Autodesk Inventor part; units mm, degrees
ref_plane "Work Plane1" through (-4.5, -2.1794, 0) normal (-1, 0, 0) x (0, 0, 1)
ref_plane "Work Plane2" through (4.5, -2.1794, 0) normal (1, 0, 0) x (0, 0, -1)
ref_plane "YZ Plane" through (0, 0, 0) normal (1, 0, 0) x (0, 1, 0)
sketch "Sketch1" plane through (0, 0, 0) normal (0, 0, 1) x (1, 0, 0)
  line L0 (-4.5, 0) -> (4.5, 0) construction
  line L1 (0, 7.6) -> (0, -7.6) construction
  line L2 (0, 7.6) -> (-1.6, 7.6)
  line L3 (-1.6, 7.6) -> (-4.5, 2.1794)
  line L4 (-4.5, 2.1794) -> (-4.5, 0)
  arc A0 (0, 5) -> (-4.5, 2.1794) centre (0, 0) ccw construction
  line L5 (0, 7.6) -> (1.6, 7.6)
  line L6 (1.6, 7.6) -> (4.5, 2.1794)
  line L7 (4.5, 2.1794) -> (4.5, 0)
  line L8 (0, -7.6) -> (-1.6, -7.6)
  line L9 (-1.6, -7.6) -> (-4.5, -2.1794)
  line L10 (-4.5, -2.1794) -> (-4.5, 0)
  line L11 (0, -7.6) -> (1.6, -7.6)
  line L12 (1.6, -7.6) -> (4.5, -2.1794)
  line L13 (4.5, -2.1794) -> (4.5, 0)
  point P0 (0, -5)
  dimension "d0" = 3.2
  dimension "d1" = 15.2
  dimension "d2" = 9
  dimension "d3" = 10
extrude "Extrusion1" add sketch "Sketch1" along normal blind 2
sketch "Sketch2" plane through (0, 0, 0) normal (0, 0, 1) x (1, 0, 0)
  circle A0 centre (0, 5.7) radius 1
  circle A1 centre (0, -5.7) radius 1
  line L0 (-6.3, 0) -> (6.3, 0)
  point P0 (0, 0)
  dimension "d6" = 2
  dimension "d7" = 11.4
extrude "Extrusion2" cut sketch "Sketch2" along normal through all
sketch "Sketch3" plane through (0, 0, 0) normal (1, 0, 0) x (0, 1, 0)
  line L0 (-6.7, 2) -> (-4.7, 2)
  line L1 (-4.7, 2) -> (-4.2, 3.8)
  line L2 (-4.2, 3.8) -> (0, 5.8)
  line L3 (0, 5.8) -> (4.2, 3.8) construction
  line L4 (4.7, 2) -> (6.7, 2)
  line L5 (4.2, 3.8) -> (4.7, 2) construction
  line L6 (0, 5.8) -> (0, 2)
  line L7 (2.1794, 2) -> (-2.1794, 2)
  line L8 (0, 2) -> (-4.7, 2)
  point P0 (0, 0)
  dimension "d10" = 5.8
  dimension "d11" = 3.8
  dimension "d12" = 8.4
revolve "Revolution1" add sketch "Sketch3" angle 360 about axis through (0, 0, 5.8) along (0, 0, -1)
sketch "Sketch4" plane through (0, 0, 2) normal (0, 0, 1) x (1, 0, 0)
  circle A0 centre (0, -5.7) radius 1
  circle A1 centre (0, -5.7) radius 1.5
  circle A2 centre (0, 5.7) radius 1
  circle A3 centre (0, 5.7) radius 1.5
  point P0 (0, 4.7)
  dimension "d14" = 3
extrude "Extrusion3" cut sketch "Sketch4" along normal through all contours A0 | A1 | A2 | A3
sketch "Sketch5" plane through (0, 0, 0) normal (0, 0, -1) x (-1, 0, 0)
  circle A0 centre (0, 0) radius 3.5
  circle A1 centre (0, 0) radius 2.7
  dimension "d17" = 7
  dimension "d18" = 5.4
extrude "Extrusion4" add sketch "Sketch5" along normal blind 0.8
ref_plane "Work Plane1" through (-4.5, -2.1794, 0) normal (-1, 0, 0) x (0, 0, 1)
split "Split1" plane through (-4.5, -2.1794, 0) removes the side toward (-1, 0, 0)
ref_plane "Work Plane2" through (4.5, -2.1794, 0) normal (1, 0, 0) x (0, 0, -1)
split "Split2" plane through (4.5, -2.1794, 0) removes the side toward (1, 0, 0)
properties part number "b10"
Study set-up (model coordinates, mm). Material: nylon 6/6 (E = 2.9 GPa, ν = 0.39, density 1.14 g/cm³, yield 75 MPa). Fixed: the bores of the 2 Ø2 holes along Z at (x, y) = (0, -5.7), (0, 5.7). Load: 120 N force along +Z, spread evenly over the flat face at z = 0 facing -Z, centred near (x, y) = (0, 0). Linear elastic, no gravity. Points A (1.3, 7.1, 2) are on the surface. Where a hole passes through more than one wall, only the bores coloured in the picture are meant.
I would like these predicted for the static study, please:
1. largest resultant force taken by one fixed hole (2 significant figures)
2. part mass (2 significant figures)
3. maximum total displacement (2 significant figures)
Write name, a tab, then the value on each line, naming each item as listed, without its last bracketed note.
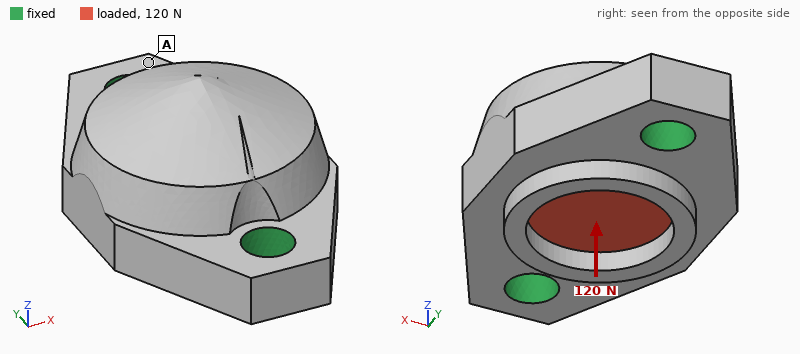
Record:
largest resultant force taken by one fixed hole	64 N
part mass	0.41 g
maximum total displacement	24 µm
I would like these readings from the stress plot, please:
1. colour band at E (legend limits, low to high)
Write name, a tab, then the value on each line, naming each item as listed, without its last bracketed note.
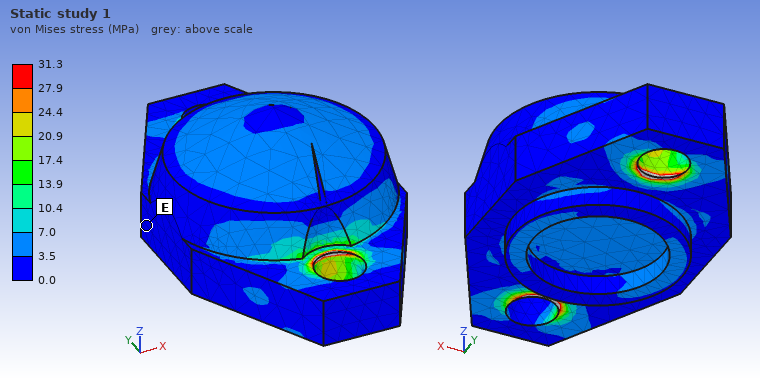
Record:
colour band at E	0.0 to 3.5 MPa
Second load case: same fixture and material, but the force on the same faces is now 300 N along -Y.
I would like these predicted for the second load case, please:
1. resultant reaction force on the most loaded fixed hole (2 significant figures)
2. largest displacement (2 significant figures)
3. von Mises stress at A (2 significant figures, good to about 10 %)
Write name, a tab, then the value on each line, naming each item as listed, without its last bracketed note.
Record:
resultant reaction force on the most loaded fixed hole	150 N
largest displacement	32 µm
von Mises stress at A	7.0 MPa
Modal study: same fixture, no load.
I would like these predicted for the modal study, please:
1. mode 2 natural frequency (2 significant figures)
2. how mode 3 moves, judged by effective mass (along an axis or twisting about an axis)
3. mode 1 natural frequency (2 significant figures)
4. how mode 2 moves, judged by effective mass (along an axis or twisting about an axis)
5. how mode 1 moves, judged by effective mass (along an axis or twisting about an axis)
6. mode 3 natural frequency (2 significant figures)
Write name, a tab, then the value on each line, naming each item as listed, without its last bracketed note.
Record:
mode 2 natural frequency	22 kHz
how mode 3 moves, judged by effective mass	along X
mode 1 natural frequency	13 kHz
how mode 2 moves, judged by effective mass	along Z
how mode 1 moves, judged by effective mass	along X
mode 3 natural frequency	28 kHz
